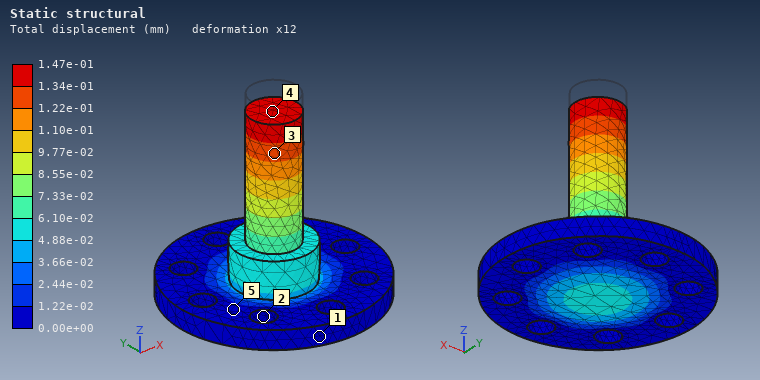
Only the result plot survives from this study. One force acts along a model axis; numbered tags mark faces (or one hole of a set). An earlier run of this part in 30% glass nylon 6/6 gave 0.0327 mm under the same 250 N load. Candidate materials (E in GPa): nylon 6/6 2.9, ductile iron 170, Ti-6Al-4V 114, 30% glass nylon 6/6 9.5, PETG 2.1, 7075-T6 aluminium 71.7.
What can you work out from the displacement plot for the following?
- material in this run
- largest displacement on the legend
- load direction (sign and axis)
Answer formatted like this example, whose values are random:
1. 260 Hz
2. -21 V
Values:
1. PETG
2. 1.47e-01 mm
3. -Z
